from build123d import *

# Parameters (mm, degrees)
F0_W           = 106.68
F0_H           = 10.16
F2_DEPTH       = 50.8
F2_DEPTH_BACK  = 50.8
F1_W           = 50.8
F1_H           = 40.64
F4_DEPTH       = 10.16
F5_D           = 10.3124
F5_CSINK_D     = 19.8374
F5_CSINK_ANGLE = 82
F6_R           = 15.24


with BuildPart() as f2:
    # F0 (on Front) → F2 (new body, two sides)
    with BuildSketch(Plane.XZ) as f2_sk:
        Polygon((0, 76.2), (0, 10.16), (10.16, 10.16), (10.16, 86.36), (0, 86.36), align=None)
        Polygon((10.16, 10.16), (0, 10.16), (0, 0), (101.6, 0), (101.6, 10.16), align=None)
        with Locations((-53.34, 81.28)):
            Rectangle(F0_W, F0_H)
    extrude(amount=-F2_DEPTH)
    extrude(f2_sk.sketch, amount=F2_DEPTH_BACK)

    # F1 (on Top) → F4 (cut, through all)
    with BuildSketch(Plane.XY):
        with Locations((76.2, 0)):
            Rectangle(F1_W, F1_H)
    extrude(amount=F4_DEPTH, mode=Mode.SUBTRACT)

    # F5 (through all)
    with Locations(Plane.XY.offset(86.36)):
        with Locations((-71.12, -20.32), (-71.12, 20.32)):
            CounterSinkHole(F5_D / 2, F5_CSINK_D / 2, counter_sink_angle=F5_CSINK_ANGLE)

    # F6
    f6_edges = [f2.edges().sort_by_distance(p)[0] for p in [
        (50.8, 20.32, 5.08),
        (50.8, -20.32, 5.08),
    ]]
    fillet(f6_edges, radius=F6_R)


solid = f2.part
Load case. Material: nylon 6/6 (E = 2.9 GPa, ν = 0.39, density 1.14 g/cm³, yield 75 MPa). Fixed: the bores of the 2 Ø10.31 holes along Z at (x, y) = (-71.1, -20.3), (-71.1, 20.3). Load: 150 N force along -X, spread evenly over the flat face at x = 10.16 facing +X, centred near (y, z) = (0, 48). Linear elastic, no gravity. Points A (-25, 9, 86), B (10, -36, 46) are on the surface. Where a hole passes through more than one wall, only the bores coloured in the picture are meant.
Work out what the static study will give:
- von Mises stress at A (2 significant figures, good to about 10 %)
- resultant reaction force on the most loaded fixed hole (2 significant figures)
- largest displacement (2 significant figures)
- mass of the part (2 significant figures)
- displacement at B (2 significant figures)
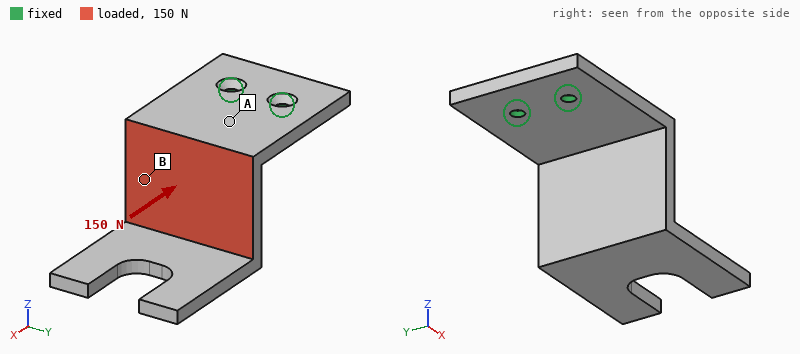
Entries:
2.3 MPa
86 N
3.0 mm
310 g
1.0 mm
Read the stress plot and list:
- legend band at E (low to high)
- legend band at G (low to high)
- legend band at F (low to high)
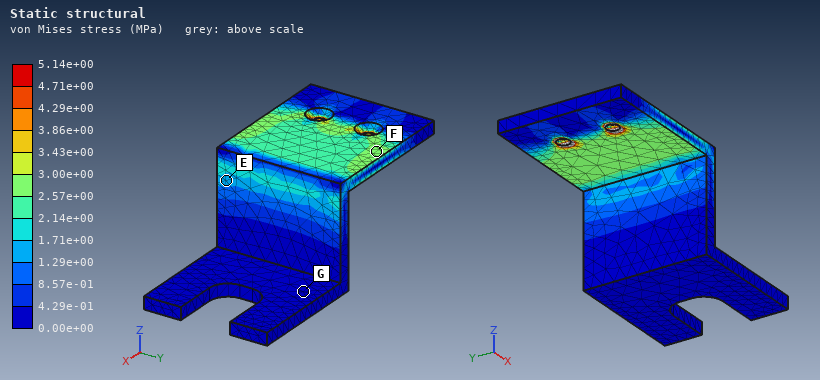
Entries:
1.29e+00 to 1.71e+00 MPa
0.00e+00 to 4.29e-01 MPa
2.57e+00 to 3.00e+00 MPa
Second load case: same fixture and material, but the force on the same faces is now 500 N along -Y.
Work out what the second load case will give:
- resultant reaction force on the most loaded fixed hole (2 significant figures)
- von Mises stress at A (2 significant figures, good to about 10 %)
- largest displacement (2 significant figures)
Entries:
920 N
5.2 MPa
2.6 mm
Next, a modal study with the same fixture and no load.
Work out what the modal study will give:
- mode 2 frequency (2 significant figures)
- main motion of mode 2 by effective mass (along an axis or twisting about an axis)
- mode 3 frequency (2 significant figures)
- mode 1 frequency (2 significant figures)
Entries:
130 Hz
along Y
240 Hz
62 Hz
